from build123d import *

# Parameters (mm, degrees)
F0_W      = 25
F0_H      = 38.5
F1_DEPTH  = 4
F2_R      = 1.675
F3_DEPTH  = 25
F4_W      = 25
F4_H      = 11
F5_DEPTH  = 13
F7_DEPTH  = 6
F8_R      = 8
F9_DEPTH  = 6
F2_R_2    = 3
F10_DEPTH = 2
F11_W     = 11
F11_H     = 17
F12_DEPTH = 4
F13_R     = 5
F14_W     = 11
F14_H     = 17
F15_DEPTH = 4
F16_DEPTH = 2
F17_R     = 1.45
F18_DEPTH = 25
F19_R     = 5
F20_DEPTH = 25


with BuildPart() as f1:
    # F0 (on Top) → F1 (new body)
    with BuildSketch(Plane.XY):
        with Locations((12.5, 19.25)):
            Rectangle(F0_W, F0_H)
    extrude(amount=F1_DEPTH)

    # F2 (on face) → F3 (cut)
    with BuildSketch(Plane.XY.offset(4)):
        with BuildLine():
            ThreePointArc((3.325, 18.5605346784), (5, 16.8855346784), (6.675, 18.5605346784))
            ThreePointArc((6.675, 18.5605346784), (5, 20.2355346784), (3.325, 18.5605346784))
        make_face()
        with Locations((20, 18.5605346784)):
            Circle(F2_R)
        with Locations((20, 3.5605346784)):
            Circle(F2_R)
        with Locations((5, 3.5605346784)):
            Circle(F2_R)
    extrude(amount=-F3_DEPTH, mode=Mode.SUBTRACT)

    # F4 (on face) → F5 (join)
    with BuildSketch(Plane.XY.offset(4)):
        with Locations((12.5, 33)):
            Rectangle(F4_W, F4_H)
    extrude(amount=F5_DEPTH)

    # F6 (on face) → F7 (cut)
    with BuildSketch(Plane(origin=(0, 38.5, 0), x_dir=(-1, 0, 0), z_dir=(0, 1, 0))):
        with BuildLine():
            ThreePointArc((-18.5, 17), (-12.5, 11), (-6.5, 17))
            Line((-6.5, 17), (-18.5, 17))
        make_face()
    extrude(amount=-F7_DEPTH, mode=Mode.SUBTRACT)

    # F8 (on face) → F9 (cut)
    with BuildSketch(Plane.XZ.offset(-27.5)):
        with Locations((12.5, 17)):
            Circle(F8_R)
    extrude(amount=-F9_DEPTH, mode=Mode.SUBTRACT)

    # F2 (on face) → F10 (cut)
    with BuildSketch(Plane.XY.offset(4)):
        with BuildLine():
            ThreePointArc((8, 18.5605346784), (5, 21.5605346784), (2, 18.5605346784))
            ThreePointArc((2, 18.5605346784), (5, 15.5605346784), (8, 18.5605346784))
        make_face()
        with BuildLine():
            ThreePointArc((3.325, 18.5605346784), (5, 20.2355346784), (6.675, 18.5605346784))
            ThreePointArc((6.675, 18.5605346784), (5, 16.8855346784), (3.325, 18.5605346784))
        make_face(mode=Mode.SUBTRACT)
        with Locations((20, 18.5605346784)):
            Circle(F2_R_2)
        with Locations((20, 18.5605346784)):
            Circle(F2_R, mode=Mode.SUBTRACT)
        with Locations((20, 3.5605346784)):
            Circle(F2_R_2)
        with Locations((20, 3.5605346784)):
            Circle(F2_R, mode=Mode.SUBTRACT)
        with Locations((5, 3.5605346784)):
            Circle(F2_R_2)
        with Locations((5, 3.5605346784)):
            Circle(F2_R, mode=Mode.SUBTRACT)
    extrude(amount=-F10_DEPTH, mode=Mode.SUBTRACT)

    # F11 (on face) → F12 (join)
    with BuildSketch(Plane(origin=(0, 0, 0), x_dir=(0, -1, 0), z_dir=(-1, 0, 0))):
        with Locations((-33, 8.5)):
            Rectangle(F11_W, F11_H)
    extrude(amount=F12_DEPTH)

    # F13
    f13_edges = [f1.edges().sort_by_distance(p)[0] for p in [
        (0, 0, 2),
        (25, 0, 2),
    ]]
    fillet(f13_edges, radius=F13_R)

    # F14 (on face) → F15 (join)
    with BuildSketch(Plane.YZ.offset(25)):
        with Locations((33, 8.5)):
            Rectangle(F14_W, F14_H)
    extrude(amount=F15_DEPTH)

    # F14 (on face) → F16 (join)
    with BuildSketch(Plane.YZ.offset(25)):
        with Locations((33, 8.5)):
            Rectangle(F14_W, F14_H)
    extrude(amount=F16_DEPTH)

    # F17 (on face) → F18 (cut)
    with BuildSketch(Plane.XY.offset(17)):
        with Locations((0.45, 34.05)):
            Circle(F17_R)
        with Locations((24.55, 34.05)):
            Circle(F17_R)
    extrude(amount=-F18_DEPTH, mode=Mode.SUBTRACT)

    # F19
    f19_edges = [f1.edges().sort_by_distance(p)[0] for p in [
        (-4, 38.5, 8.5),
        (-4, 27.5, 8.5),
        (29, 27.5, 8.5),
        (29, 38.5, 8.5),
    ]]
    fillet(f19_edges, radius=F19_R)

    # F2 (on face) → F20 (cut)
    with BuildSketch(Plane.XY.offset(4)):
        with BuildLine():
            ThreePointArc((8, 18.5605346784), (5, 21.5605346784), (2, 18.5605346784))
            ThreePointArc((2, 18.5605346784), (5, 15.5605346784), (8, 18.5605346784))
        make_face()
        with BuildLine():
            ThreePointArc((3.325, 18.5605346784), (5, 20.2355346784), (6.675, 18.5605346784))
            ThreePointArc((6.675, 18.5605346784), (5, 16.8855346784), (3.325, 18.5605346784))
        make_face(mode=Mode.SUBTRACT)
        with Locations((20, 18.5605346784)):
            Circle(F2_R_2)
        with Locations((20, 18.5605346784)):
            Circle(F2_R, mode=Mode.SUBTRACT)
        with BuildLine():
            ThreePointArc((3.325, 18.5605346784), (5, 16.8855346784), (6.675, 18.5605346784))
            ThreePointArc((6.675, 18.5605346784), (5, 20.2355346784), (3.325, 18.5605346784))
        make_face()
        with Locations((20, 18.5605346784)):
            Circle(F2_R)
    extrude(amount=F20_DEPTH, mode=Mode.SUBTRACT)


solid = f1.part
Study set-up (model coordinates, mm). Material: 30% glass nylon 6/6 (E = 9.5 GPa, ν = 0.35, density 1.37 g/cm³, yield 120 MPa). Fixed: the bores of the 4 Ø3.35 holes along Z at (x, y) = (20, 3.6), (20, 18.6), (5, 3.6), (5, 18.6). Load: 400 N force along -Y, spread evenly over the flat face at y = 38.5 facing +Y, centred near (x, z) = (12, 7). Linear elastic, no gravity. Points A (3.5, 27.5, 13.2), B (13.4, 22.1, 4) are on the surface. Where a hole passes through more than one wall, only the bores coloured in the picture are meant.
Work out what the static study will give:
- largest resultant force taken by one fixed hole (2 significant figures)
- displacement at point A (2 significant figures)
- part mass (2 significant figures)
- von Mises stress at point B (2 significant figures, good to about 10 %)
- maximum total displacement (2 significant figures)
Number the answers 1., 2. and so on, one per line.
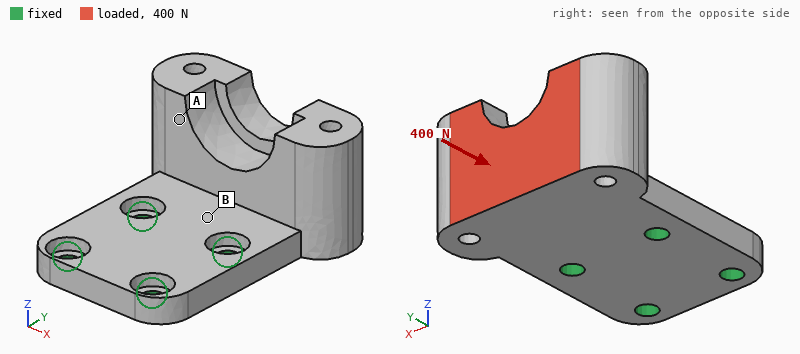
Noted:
1. 150 N
2. 0.31 mm
3. 9.7 g
4. 41 MPa
5. 0.55 mm
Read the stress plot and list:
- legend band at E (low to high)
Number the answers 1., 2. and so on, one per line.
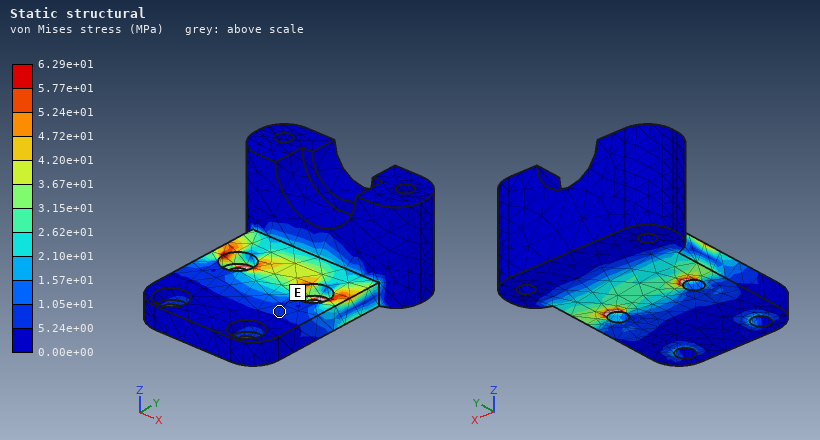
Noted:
1. 5.24e+00 to 1.05e+01 MPa
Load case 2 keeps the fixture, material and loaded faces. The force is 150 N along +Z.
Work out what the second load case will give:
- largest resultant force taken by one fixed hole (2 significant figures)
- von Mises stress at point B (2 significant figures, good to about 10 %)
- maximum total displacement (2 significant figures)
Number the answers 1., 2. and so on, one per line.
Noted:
1. 180 N
2. 40 MPa
3. 0.56 mm
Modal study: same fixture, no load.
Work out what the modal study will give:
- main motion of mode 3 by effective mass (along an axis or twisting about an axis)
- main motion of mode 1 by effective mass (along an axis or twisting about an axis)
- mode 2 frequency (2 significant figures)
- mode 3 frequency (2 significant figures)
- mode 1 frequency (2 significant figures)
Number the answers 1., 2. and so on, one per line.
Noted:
1. along X
2. along Z
3. 3200 Hz
4. 6400 Hz
5. 1400 Hz
